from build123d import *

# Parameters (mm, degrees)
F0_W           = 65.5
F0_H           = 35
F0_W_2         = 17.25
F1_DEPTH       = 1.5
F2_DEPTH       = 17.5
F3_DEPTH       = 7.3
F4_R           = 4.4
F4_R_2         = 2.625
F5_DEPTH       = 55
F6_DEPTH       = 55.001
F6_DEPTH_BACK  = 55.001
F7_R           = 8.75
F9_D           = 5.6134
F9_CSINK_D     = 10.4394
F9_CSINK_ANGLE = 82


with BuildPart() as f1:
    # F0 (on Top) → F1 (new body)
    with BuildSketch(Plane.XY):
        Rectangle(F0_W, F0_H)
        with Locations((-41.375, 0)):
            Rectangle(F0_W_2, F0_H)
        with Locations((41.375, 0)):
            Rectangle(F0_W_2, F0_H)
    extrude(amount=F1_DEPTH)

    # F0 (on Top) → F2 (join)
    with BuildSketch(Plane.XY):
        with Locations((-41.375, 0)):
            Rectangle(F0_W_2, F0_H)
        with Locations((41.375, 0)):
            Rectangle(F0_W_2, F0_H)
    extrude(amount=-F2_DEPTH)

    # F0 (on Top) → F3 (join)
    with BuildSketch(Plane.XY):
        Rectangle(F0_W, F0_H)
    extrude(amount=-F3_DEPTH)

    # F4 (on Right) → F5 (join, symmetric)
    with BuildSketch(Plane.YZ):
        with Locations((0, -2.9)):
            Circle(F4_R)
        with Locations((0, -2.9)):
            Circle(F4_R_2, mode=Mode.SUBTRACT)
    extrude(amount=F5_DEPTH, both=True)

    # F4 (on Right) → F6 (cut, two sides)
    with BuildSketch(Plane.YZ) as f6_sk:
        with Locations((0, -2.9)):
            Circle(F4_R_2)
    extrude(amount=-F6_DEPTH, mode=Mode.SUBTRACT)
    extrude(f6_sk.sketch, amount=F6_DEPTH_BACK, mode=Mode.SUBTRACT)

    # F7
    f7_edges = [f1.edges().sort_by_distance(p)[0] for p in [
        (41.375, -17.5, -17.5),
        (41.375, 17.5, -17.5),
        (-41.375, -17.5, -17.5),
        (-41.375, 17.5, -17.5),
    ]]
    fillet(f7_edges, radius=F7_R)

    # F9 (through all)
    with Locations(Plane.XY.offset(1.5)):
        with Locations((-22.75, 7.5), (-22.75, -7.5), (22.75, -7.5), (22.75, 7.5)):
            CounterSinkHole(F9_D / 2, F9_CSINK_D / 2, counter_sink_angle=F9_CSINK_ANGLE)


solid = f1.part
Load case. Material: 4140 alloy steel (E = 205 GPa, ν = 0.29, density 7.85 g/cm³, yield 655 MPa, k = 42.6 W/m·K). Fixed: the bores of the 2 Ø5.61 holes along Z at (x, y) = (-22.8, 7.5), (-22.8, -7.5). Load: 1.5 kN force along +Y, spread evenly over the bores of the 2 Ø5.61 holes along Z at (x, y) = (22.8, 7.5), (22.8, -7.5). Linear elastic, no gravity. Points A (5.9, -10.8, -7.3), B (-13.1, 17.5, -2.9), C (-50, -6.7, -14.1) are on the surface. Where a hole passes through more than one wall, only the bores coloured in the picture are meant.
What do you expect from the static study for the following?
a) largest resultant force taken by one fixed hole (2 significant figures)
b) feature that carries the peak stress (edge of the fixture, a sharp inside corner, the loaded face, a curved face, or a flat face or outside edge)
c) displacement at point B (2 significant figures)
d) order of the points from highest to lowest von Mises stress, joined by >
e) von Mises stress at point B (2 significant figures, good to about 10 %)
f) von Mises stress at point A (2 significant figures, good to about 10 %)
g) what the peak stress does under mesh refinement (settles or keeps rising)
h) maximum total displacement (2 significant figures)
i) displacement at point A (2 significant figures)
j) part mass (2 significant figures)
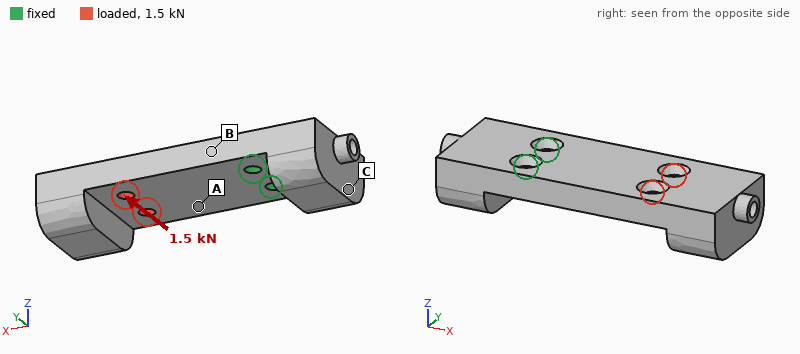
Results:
3.5 kN
edge of the fixture
4.4 µm
B > A > C
27 MPa
16 MPa
keeps rising
28 µm
9.8 µm
310 g
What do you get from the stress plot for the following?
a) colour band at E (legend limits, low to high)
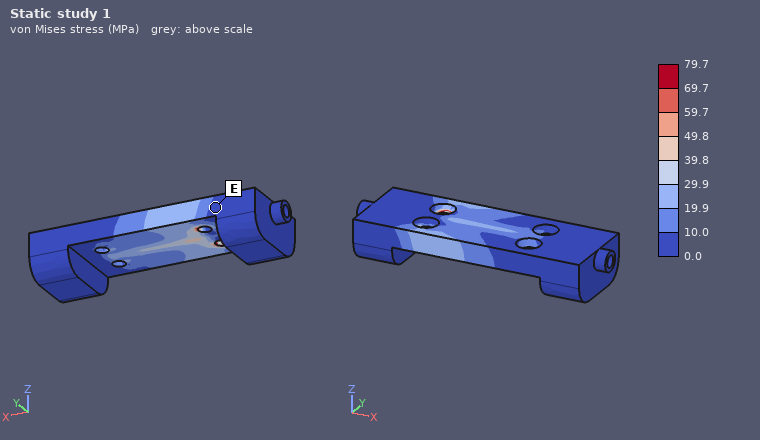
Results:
0.0 to 10.0 MPa
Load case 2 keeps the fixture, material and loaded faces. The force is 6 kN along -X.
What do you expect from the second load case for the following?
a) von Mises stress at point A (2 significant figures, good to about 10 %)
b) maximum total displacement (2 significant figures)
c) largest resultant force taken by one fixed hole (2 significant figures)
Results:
39 MPa
49 µm
3.0 kN
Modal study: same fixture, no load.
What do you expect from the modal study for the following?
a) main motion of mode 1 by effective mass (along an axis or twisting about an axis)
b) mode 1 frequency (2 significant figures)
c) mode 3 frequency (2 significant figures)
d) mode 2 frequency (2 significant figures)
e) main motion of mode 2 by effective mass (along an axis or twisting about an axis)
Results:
along Z
970 Hz
4200 Hz
2900 Hz
along Y
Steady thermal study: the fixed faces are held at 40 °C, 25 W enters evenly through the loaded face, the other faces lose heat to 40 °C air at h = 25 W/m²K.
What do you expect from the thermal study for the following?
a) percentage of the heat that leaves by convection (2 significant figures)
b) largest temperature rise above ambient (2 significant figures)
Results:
39 %
69 K
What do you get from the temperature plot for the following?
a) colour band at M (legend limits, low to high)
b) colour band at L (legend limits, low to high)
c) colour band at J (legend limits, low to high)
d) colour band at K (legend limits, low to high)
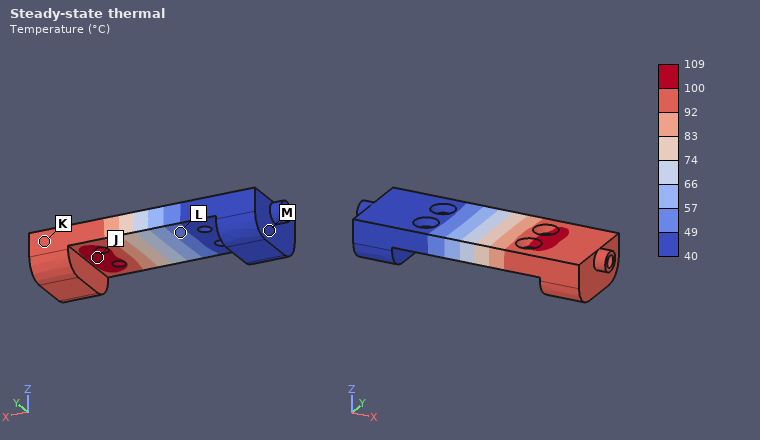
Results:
40 to 49 °C
49 to 57 °C
100 to 109 °C
92 to 100 °C
